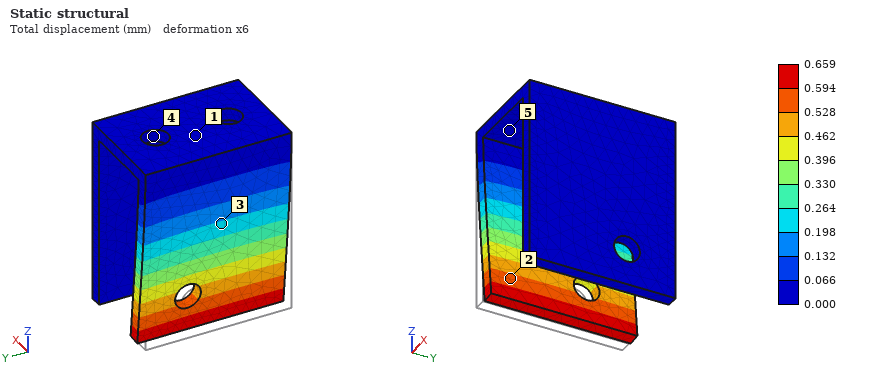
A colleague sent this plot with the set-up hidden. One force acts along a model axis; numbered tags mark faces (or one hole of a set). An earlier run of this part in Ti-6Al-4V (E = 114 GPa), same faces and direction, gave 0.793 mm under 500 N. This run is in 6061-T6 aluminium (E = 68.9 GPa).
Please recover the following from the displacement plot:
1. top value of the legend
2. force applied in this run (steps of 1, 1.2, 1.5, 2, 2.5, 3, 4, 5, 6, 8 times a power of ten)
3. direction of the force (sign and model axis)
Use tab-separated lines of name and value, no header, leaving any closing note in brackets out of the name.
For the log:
top value of the legend	0.659 mm
force applied in this run	250 N
direction of the force	+X
